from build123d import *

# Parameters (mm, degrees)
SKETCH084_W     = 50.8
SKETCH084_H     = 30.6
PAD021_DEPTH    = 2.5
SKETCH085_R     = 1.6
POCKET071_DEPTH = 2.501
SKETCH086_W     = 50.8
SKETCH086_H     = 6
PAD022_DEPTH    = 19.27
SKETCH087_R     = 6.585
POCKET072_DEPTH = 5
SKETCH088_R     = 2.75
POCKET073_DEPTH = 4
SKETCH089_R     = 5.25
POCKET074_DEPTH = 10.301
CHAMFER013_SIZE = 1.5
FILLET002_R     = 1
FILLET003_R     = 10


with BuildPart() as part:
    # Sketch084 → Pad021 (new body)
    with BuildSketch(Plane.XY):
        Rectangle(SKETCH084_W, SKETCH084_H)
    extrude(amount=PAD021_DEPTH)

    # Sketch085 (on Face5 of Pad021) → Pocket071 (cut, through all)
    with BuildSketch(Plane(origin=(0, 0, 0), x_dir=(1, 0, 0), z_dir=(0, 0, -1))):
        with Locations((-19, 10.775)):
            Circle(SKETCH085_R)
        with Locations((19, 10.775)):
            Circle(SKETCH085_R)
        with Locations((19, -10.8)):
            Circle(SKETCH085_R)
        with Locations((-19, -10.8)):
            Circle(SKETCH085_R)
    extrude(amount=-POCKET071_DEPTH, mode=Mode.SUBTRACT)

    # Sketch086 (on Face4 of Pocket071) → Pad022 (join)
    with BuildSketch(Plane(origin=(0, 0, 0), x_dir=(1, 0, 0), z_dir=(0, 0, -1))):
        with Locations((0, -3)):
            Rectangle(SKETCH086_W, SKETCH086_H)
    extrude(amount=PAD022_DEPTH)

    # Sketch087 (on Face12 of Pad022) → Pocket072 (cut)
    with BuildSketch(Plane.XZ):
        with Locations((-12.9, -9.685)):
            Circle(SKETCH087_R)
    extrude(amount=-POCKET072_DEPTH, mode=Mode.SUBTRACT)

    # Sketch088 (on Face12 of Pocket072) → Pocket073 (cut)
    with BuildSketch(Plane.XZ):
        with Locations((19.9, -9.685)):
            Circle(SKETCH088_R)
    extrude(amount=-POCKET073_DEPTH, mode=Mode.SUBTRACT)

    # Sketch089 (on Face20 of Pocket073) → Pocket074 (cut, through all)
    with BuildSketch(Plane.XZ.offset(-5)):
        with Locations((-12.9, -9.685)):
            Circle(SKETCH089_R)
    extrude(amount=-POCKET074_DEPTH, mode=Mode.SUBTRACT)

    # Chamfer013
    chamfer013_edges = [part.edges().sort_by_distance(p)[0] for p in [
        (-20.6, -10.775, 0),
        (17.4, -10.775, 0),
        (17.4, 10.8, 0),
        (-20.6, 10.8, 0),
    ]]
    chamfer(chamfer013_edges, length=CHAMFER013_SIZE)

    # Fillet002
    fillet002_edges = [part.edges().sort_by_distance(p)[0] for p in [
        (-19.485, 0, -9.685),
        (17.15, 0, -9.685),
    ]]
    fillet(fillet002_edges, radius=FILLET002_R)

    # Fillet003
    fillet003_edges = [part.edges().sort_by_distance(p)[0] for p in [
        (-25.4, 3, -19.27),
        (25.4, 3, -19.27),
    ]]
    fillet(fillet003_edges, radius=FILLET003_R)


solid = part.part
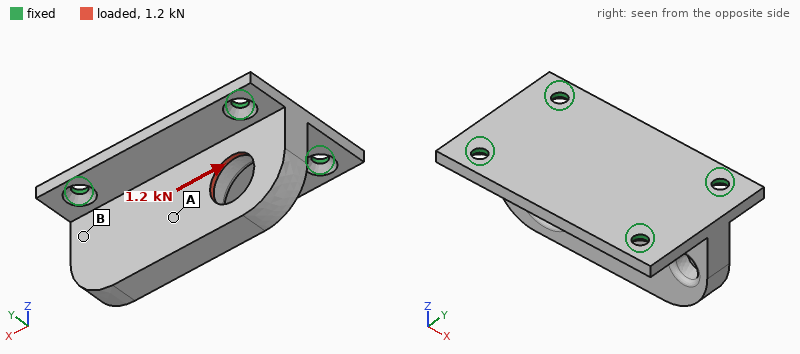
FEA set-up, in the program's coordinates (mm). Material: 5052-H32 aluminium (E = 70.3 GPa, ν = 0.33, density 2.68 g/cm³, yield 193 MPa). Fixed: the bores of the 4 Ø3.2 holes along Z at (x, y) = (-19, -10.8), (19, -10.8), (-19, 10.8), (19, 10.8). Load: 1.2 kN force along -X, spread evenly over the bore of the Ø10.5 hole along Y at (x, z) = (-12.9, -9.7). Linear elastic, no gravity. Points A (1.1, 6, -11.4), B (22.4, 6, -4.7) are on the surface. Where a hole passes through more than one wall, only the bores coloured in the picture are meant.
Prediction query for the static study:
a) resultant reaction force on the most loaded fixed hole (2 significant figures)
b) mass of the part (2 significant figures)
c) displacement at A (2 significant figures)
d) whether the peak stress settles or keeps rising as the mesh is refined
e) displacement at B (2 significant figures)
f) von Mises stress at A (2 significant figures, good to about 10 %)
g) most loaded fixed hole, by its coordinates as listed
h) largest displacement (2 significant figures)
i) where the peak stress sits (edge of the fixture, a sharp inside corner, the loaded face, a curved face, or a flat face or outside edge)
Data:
560 N
23 g
13 µm
keeps rising
13 µm
17 MPa
(-19, 10.8)
29 µm
edge of the fixture
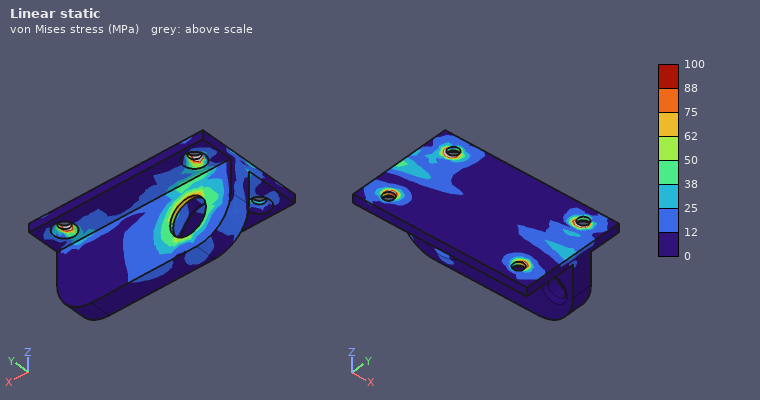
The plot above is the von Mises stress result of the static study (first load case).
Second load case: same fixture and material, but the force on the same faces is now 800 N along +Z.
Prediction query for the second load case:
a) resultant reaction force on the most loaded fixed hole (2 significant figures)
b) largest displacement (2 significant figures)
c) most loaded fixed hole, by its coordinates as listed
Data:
630 N
24 µm
(-19, 10.8)
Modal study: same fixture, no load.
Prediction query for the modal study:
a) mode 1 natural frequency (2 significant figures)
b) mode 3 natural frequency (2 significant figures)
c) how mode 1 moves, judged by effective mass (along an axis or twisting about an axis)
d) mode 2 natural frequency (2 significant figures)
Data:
5400 Hz
10000 Hz
along Y
9800 Hz
